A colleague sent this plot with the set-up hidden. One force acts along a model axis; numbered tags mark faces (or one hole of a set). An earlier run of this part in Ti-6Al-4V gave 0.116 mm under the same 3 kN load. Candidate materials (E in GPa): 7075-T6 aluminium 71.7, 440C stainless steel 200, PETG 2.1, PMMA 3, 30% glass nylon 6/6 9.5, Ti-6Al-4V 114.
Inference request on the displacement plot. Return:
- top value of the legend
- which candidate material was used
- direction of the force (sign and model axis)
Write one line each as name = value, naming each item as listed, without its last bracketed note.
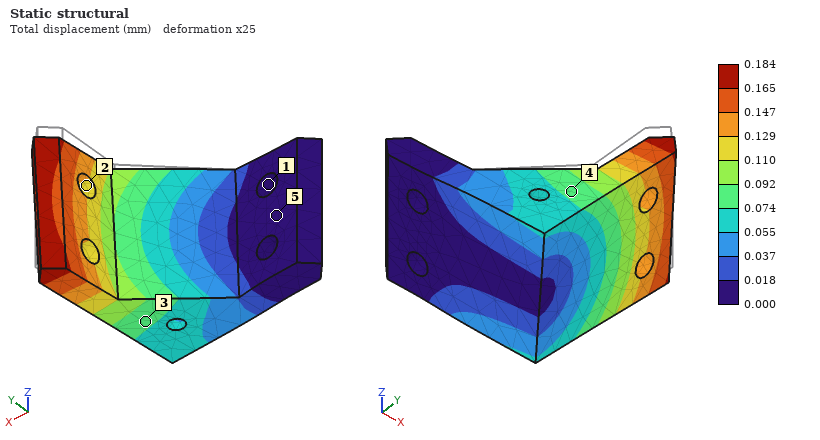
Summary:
top value of the legend = 0.184 mm
which candidate material was used = 7075-T6 aluminium
direction of the force = -Z
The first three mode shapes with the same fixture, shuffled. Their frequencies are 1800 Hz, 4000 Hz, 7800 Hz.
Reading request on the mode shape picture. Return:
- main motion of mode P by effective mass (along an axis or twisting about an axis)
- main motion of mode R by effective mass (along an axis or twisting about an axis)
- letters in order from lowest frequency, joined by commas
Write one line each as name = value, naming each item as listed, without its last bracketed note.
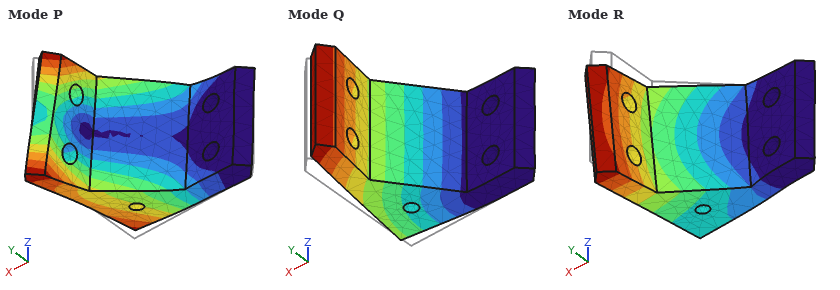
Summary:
main motion of mode P by effective mass = along Z
main motion of mode R by effective mass = along Z
letters in order from lowest frequency, joined by commas = Q, R, P
